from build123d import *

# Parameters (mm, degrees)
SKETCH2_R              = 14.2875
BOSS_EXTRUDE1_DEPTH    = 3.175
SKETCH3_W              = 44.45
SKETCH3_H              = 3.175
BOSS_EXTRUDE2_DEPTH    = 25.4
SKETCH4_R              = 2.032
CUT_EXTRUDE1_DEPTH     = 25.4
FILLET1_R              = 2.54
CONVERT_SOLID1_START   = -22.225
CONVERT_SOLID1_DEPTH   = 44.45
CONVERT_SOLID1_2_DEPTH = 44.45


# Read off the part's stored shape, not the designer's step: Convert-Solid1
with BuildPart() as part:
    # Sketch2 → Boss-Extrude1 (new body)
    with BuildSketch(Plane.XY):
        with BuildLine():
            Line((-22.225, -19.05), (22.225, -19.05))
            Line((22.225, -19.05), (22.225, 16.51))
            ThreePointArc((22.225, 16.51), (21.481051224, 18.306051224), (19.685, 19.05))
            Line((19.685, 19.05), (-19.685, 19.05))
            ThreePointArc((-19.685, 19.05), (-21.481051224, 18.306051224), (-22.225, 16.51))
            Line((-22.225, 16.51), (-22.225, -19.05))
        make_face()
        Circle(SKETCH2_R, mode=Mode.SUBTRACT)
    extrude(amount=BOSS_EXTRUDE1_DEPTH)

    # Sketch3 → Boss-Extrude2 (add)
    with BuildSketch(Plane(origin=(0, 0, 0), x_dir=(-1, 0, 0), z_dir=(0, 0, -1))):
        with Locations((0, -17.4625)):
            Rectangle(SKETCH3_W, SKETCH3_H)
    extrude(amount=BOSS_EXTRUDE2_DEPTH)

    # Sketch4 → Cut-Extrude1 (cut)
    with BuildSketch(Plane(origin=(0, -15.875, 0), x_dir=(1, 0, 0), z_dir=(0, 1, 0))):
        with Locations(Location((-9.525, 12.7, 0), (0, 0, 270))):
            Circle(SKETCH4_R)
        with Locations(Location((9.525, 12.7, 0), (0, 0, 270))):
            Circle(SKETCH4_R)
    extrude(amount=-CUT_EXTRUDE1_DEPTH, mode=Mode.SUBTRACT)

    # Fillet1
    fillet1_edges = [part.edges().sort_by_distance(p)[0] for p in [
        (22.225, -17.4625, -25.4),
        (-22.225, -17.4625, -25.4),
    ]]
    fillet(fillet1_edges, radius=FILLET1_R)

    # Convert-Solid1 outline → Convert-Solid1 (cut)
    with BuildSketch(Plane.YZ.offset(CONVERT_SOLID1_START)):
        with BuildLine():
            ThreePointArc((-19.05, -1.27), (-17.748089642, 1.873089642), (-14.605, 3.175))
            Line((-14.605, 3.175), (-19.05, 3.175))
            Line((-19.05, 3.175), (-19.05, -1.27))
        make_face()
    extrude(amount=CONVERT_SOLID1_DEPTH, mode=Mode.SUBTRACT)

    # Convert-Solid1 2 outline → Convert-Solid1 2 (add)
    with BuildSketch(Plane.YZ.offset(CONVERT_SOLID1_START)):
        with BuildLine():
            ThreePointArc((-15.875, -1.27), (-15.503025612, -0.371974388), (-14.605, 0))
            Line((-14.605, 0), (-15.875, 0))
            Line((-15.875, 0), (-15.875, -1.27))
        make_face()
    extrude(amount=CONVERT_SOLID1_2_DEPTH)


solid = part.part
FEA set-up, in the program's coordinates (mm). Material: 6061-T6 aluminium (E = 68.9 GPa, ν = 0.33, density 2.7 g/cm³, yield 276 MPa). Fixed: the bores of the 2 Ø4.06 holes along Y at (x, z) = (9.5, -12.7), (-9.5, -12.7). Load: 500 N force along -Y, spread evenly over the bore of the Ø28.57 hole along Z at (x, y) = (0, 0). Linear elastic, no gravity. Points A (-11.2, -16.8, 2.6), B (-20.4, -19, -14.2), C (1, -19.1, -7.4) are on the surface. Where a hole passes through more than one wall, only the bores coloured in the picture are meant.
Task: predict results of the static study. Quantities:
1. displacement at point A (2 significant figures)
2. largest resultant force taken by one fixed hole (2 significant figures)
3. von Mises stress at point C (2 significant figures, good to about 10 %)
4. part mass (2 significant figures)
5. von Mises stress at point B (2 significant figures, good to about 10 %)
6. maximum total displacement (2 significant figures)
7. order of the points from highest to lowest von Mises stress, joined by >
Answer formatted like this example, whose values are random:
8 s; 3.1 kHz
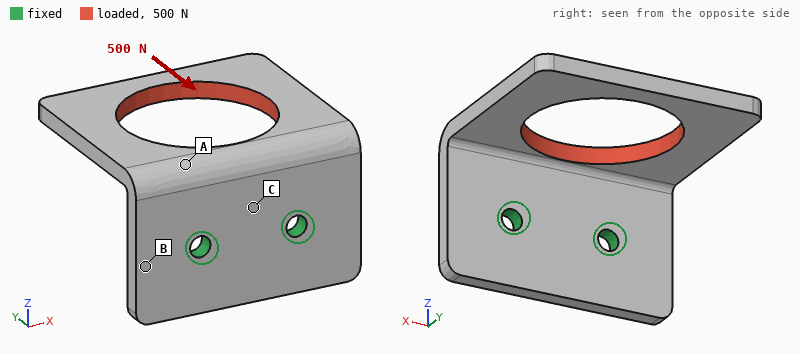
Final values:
0.068 mm; 250 N; 47 MPa; 18 g; 27 MPa; 0.24 mm; C > B > A
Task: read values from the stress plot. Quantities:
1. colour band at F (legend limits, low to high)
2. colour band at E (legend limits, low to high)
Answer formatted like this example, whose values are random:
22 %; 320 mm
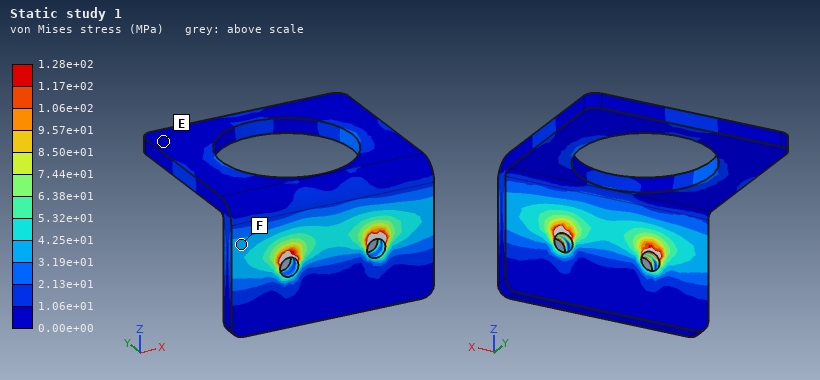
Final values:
3.19e+01 to 4.25e+01 MPa; 0.00e+00 to 1.06e+01 MPa
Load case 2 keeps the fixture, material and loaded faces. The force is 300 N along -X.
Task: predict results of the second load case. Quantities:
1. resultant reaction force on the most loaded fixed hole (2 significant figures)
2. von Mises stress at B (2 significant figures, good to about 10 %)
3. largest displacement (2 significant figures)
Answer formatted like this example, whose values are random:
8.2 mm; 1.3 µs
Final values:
310 N; 23 MPa; 0.14 mm
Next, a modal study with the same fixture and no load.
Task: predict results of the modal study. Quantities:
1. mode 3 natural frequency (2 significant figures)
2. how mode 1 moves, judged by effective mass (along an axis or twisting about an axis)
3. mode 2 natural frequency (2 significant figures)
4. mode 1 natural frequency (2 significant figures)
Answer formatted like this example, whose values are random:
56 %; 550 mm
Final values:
3400 Hz; along Z; 2400 Hz; 1200 Hz
